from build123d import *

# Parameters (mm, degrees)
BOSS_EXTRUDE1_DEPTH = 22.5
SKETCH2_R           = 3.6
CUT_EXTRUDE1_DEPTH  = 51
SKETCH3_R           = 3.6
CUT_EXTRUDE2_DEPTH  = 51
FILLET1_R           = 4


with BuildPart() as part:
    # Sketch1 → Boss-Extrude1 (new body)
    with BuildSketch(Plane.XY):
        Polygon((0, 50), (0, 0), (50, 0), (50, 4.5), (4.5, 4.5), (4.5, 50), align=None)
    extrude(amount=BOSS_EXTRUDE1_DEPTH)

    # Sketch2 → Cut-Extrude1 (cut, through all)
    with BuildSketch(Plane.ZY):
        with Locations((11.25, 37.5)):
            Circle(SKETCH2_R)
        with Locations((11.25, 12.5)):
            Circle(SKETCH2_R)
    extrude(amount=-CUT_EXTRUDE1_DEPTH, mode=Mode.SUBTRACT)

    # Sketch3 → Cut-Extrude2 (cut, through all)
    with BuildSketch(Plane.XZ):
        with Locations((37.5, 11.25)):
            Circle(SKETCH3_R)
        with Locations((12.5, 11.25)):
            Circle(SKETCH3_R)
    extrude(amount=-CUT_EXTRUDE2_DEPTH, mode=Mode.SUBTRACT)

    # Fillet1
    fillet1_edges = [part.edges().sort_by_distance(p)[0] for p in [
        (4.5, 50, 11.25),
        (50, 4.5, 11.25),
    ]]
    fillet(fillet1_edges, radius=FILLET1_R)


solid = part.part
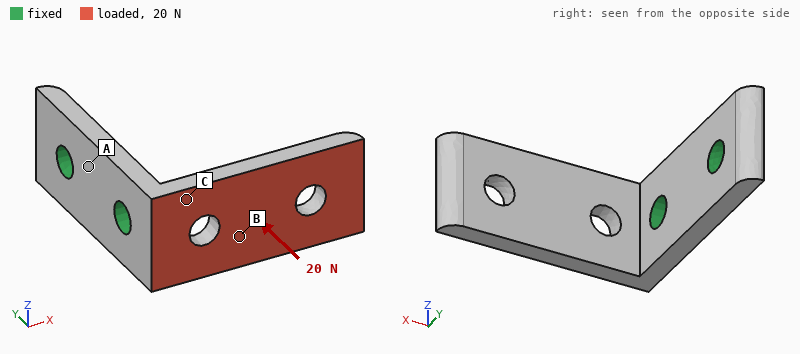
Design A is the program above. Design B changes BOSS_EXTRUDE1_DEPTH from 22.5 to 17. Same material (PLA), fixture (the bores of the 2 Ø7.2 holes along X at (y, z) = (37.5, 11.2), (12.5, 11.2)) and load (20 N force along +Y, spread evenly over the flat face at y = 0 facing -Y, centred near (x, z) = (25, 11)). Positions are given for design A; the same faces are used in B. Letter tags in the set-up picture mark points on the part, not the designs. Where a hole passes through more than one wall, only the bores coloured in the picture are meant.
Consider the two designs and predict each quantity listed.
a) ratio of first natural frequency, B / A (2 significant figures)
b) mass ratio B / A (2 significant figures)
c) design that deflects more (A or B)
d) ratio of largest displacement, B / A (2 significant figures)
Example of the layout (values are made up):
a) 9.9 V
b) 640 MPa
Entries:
a) 0.98
b) 0.74
c) B
d) 1.4
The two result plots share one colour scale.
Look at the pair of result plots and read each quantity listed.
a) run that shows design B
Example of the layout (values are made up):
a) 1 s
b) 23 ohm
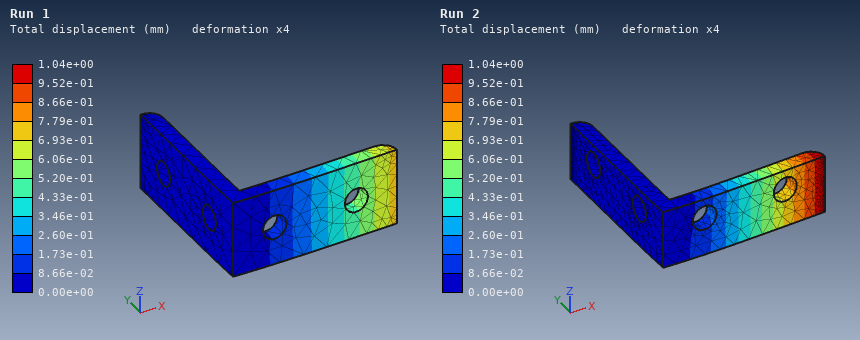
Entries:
a) Run 2
